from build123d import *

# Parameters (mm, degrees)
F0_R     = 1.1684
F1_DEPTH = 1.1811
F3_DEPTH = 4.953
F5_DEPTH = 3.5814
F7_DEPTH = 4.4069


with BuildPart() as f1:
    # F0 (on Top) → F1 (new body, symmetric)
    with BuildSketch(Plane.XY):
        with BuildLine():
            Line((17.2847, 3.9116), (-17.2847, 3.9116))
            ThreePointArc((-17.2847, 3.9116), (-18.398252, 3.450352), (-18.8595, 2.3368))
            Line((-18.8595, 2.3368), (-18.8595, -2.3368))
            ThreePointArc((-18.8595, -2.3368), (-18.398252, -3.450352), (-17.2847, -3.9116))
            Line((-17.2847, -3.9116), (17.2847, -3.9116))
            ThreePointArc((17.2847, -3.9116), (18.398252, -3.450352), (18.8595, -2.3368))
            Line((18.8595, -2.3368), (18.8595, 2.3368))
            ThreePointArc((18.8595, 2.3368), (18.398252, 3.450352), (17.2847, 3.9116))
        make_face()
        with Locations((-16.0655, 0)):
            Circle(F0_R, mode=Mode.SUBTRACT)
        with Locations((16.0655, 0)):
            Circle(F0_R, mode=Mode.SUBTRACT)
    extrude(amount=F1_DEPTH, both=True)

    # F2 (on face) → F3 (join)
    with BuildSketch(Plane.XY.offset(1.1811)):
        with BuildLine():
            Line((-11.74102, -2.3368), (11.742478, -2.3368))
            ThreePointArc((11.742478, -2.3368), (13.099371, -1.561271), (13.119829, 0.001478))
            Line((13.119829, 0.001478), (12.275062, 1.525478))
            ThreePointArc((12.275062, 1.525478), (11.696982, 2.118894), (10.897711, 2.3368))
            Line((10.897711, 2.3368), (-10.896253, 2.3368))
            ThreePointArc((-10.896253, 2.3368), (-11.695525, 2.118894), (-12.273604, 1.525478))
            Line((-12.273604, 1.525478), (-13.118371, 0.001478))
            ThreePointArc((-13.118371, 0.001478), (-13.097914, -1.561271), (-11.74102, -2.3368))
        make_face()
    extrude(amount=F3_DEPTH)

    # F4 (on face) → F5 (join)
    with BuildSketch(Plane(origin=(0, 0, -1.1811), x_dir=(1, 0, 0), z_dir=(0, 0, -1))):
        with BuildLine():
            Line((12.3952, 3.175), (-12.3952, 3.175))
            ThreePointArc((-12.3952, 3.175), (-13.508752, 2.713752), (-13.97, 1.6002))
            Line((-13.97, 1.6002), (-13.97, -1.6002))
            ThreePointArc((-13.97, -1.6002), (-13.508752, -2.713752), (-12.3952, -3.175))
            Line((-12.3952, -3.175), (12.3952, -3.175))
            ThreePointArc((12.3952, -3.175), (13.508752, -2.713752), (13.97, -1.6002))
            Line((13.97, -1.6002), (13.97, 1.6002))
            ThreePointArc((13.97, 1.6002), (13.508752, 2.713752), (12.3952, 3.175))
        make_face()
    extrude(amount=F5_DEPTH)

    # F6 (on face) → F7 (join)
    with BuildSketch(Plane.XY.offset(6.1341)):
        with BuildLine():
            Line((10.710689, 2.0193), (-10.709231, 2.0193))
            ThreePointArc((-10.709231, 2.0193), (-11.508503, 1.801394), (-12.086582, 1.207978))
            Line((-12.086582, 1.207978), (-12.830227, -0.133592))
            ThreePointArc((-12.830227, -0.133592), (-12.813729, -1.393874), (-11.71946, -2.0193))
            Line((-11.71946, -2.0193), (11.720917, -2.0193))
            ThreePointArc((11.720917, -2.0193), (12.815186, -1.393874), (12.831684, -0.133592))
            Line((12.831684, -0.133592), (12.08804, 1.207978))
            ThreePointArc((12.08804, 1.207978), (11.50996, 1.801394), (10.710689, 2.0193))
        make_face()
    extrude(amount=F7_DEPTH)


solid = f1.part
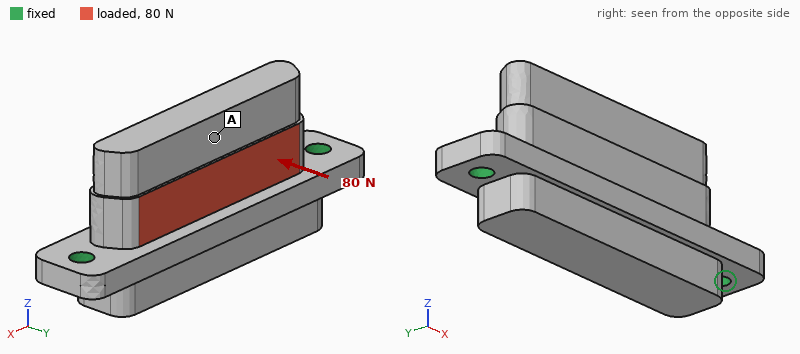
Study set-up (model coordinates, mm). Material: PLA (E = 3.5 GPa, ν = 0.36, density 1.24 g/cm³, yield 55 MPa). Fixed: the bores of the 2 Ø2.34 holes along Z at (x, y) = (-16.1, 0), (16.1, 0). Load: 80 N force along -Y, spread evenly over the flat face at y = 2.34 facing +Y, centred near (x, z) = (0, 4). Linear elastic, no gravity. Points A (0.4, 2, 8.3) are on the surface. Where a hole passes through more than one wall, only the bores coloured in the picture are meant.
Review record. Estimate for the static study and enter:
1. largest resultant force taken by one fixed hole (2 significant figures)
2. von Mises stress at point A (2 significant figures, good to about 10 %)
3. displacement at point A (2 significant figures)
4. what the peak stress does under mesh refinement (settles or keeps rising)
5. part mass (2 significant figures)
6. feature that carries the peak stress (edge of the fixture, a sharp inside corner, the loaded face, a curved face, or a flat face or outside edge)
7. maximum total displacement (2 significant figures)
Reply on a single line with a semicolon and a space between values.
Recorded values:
40 N; 2.7 MPa; 0.14 mm; keeps rising; 2.9 g; edge of the fixture; 0.16 mm
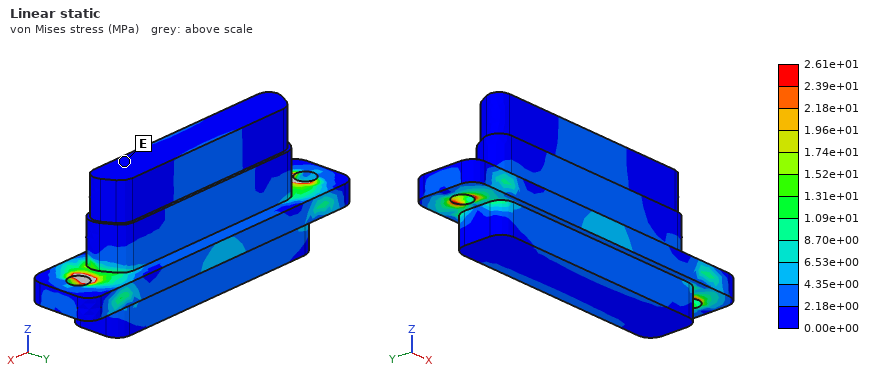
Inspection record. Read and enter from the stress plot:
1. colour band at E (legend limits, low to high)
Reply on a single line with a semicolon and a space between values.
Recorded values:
0.00e+00 to 2.18e+00 MPa
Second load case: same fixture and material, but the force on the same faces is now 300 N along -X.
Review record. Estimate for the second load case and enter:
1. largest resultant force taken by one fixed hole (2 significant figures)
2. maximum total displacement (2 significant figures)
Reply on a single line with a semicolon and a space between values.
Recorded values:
160 N; 42 µm
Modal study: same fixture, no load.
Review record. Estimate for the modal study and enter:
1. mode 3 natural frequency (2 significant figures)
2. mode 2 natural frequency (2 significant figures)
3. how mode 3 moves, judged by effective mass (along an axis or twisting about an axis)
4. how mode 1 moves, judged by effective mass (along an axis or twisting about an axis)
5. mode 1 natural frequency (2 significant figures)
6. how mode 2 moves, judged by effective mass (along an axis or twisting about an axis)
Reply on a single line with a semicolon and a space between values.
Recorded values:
6800 Hz; 5800 Hz; along Z; along Y; 3100 Hz; along Y
